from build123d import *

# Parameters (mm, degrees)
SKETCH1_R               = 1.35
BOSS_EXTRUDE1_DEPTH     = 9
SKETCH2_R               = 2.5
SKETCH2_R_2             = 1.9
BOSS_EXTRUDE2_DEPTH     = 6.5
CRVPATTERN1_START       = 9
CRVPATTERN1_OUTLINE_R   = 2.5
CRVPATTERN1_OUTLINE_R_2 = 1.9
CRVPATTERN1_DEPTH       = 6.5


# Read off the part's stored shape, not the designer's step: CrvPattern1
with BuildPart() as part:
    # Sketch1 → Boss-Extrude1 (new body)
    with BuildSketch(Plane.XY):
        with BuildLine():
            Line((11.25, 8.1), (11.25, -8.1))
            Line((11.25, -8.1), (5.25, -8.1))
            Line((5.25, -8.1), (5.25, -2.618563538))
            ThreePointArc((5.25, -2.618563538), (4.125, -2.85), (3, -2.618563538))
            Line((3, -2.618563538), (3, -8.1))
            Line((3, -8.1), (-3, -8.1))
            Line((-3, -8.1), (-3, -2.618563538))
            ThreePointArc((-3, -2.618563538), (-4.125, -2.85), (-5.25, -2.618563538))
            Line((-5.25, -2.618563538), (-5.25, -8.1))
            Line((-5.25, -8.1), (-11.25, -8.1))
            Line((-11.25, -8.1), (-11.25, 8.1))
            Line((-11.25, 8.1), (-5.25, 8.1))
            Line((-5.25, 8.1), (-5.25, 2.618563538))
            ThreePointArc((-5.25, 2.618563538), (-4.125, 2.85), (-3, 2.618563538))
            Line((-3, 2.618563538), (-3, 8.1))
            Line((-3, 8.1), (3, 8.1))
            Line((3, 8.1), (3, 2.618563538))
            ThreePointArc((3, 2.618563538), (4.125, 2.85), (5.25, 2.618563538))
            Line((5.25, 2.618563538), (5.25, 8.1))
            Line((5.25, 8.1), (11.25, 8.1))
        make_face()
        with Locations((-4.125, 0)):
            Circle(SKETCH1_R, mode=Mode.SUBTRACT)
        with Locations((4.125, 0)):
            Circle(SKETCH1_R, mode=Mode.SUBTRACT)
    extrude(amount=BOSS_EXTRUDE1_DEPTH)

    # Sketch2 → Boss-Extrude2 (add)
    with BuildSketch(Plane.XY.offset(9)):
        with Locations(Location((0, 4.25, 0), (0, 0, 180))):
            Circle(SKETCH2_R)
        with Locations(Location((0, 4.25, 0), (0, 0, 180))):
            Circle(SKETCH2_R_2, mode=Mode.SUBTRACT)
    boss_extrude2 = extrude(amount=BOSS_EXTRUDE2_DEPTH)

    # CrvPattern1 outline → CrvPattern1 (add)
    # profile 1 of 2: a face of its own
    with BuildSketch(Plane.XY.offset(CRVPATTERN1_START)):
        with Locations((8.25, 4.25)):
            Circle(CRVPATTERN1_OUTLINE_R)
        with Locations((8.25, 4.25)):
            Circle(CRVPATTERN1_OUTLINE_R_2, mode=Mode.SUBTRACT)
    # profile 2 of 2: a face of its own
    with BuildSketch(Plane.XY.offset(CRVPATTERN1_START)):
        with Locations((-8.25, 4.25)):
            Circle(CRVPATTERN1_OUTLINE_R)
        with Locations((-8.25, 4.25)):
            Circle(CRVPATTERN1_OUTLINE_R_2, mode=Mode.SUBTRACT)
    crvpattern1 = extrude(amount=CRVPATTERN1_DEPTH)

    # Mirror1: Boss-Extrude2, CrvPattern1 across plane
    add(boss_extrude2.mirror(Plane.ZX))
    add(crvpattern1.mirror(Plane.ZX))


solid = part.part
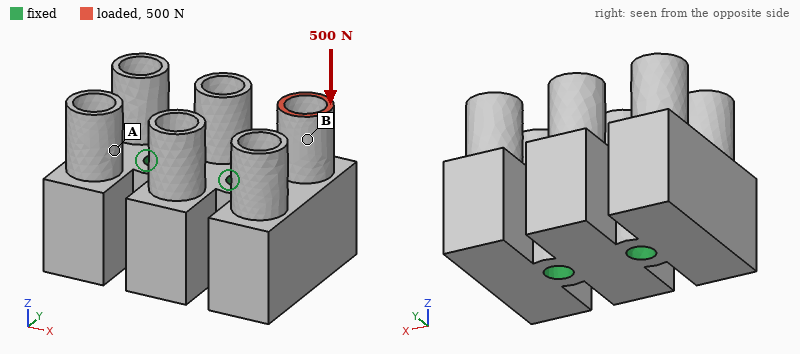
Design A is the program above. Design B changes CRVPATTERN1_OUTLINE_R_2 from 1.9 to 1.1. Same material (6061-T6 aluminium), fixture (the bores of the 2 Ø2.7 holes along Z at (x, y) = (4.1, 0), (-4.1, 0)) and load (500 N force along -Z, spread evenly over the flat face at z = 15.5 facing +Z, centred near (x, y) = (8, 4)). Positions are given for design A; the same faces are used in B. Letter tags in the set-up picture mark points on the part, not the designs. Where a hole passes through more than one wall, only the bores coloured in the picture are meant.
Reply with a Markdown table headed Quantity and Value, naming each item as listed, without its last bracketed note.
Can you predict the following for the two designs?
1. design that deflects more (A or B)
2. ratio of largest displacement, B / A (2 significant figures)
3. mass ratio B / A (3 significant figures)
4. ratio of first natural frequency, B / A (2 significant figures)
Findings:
| Quantity | Value |
|---|---|
| design that deflects more | A |
| ratio of largest displacement, B / A | 0.81 |
| mass ratio B / A | 1.06 |
| ratio of first natural frequency, B / A | 0.94 |
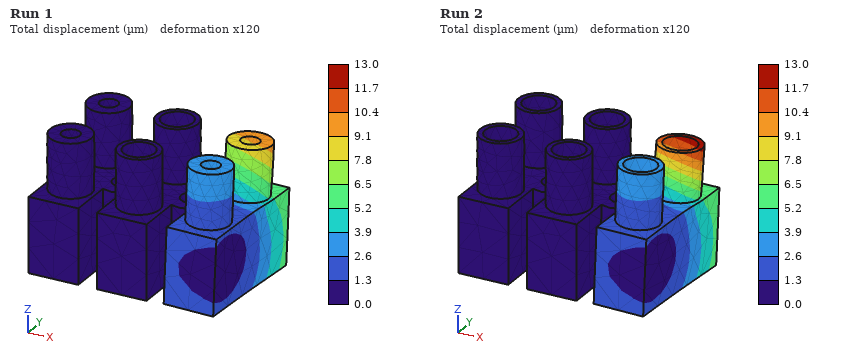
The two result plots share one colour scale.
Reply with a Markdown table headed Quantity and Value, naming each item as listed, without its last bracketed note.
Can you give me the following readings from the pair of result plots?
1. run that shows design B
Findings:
| Quantity | Value |
|---|---|
| run that shows design B | Run 1 |
